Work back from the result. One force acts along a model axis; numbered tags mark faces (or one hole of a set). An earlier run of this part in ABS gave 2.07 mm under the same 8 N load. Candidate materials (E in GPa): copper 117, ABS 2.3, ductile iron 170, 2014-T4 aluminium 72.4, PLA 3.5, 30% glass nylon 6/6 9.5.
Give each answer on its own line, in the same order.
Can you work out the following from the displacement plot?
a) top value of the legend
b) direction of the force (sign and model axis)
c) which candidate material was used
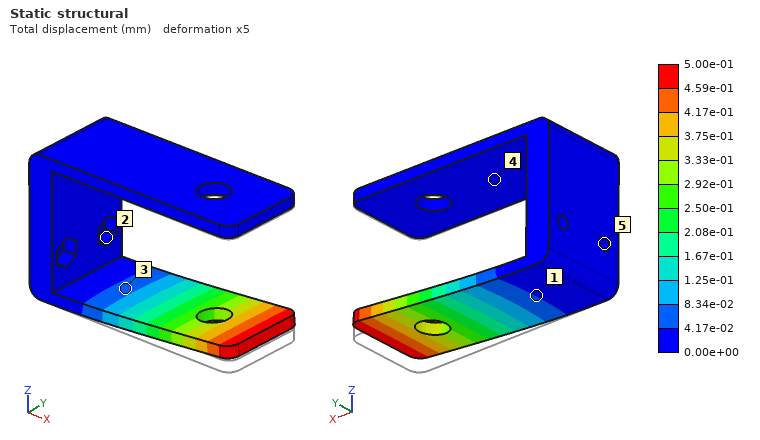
5.00e-01 mm
+Z
30% glass nylon 6/6
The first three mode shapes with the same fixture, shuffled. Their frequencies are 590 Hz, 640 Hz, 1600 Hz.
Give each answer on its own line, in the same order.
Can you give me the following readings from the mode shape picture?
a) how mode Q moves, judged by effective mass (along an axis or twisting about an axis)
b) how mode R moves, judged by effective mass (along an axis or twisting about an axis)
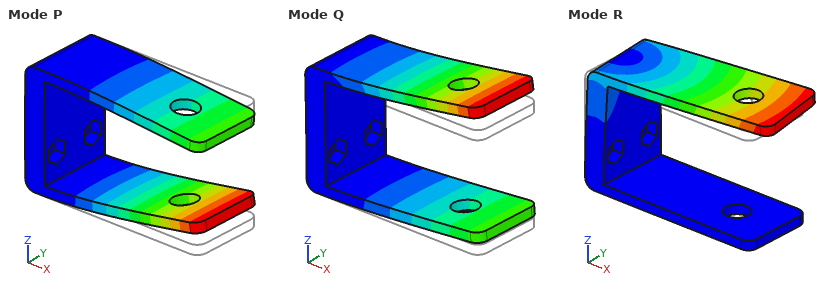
along Z
along Y
